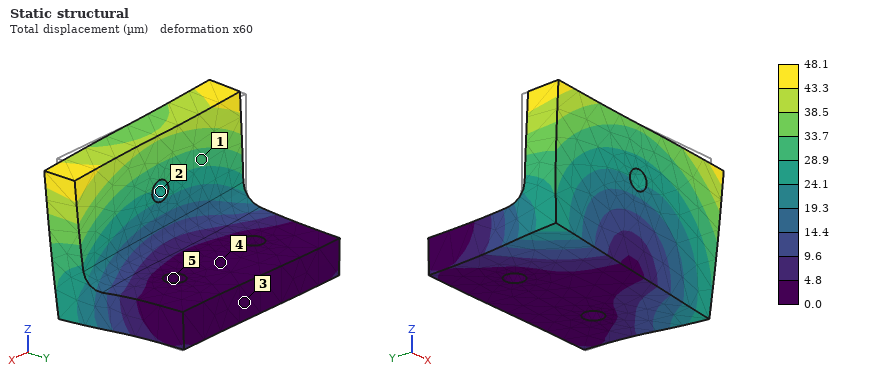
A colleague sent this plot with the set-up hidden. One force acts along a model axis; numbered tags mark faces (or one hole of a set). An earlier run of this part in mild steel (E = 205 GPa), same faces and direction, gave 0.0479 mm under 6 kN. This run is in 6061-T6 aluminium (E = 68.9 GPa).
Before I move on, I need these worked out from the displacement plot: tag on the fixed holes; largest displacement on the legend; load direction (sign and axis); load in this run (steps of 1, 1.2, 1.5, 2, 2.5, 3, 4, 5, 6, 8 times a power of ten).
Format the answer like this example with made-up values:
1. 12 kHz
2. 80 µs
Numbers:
1. 5
2. 48.1 µm
3. +X
4. 2 kN
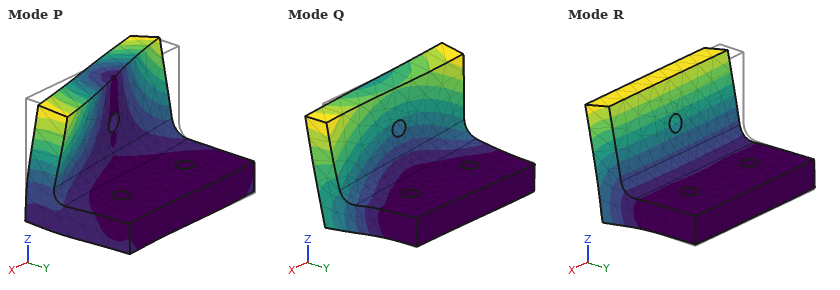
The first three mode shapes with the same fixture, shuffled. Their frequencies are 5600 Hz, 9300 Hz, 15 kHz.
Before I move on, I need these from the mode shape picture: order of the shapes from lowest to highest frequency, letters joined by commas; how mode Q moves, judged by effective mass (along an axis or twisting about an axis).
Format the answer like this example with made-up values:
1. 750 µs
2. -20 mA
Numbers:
1. R, Q, P
2. along X
